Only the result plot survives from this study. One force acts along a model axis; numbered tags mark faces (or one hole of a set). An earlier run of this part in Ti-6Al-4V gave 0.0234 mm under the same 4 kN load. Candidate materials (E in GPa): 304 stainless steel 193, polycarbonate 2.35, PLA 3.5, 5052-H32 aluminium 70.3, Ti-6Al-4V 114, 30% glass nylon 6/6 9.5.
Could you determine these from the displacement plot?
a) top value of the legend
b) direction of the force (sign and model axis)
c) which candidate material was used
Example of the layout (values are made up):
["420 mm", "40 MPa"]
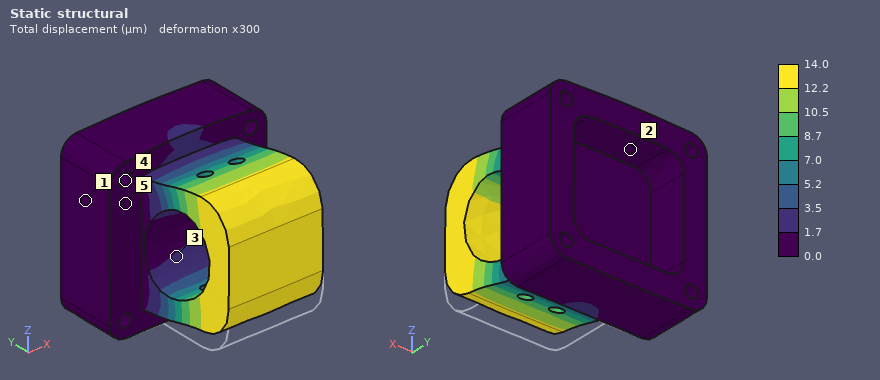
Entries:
["14.0 µm", "+Z", "304 stainless steel"]
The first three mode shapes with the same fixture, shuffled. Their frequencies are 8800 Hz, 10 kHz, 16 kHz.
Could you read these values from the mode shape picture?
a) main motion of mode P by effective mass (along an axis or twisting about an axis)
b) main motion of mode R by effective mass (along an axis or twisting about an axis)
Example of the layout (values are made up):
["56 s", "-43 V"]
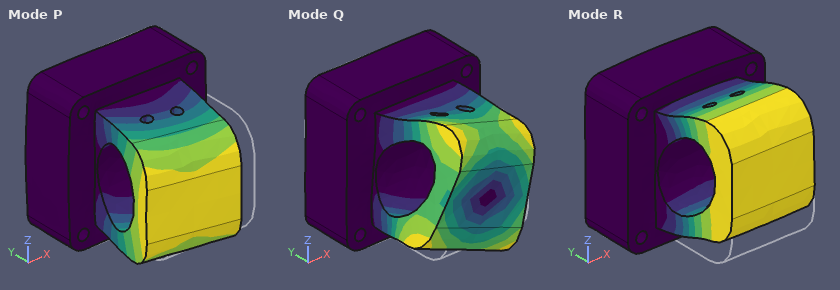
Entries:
["along X", "along Z"]
